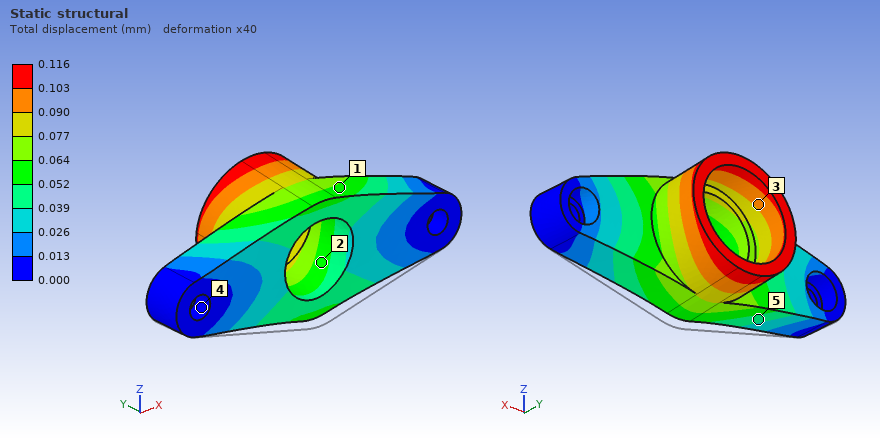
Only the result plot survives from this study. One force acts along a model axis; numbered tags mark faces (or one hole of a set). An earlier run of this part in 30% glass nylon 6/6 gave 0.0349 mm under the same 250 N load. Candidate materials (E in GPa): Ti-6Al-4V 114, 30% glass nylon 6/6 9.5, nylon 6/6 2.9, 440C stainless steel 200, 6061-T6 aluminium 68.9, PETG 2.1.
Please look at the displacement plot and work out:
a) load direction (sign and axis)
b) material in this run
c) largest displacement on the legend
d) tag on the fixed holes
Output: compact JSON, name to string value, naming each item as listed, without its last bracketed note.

{"load direction": "+Z", "material in this run": "nylon 6/6", "largest displacement on the legend": "0.116 mm", "tag on the fixed holes": "4"}
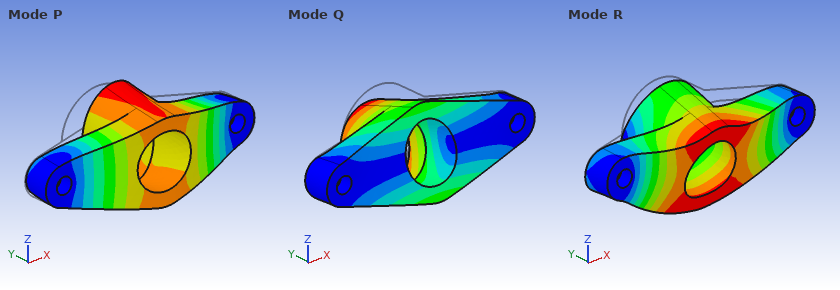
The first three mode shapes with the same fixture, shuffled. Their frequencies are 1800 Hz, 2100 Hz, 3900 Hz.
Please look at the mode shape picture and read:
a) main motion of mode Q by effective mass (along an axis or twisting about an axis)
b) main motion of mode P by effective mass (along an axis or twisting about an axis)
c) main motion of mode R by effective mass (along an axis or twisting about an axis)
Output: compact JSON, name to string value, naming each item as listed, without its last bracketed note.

{"main motion of mode Q by effective mass": "along Z", "main motion of mode P by effective mass": "along Y", "main motion of mode R by effective mass": "along Z"}
